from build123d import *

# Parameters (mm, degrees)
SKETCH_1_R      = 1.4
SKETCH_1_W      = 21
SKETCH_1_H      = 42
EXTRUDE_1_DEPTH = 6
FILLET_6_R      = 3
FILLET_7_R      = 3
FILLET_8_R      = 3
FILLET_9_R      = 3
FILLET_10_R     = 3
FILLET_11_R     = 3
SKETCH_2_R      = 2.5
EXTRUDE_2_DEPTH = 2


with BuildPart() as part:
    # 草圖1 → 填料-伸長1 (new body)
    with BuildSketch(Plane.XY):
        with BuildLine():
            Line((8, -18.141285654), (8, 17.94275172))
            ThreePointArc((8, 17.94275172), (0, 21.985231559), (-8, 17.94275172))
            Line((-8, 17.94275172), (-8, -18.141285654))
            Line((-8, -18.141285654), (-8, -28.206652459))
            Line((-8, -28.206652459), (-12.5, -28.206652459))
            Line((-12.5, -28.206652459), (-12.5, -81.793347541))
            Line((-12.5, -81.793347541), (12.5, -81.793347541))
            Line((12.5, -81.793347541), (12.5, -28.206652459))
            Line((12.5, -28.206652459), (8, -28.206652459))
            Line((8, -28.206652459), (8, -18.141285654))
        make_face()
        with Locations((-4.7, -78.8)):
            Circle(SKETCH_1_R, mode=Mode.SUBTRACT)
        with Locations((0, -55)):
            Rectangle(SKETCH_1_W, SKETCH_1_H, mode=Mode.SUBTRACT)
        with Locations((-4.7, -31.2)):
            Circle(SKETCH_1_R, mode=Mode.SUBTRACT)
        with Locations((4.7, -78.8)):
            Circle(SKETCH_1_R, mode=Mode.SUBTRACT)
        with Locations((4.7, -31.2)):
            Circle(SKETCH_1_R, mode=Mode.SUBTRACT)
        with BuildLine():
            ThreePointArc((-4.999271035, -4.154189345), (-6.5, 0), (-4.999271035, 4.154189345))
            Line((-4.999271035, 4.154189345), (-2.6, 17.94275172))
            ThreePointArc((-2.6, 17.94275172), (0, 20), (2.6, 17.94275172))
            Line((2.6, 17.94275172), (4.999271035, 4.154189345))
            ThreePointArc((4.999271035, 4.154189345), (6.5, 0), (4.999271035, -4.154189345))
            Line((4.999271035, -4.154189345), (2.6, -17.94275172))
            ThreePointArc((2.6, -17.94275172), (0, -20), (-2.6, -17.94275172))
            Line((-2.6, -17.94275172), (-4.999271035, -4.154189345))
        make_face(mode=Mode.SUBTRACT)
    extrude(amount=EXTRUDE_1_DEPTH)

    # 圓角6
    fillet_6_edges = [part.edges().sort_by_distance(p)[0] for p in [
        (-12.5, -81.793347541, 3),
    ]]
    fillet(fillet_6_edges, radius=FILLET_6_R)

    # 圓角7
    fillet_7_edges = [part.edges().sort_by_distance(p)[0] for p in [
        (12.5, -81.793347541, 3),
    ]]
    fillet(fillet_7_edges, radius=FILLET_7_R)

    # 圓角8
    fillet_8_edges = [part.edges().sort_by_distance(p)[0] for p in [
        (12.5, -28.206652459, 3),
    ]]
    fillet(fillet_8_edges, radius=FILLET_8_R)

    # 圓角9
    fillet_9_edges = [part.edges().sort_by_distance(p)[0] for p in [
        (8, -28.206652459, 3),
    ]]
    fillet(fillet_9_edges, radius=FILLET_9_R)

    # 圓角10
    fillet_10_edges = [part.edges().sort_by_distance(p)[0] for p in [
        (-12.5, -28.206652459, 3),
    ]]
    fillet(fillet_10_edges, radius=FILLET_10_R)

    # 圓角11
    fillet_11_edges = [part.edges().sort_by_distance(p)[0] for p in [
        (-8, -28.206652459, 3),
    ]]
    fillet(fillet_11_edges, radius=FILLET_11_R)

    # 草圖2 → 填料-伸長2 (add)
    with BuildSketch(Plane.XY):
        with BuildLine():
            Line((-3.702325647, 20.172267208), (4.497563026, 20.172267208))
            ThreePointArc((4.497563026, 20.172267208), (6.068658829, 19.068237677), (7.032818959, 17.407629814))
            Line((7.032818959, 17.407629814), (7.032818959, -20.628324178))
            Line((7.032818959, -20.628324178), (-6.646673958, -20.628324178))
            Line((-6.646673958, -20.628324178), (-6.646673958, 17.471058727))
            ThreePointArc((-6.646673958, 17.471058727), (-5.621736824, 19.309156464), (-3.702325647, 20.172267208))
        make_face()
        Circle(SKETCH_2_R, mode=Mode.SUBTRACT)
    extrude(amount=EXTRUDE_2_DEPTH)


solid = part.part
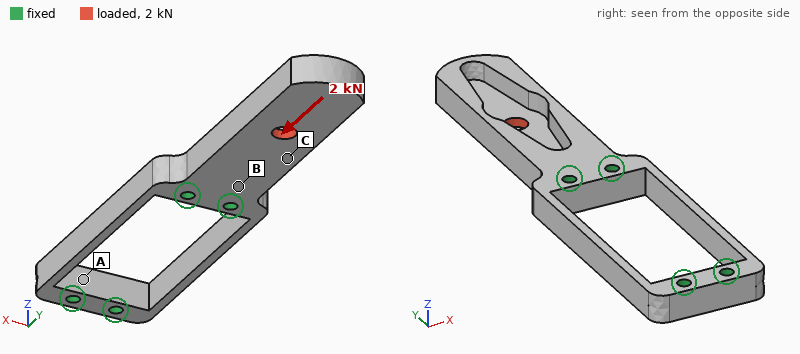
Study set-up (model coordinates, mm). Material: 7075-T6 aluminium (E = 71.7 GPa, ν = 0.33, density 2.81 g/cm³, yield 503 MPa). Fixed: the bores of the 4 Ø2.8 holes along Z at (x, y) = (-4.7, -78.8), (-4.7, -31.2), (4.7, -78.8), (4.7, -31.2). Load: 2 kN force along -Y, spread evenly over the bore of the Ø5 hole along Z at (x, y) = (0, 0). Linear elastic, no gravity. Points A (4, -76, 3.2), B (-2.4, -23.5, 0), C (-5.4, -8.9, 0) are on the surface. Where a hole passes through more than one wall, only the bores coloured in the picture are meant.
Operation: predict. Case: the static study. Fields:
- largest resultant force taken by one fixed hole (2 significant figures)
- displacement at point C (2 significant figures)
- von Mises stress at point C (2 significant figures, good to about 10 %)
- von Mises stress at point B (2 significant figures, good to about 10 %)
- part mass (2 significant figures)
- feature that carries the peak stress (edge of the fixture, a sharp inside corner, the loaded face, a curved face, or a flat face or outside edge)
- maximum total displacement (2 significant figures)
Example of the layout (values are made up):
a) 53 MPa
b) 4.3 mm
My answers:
a) 1000 N
b) 0.050 mm
c) 68 MPa
d) 59 MPa
e) 17 g
f) the loaded face
g) 0.23 mm
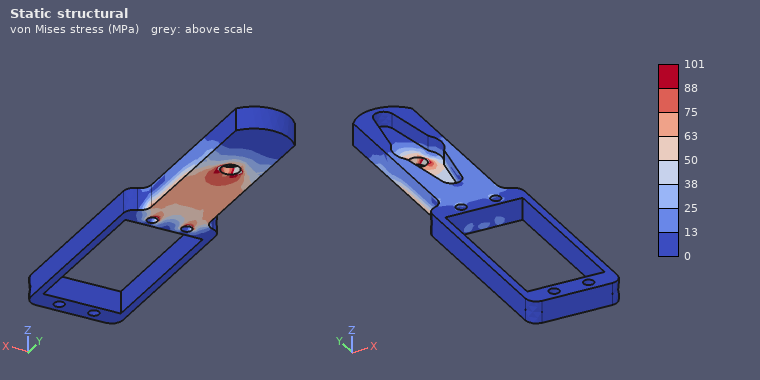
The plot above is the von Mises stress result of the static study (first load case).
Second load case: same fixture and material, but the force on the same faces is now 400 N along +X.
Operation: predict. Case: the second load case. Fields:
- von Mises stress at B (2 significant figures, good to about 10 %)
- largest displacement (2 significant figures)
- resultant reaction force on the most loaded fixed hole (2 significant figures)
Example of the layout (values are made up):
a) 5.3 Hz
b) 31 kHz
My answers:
a) 17 MPa
b) 82 µm
c) 1.1 kN
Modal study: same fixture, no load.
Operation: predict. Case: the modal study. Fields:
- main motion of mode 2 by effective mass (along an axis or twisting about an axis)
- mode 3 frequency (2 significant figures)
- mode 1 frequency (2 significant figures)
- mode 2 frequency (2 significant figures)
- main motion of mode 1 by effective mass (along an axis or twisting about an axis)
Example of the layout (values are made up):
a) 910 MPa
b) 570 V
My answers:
a) along X
b) 5300 Hz
c) 2000 Hz
d) 4400 Hz
e) along Z
